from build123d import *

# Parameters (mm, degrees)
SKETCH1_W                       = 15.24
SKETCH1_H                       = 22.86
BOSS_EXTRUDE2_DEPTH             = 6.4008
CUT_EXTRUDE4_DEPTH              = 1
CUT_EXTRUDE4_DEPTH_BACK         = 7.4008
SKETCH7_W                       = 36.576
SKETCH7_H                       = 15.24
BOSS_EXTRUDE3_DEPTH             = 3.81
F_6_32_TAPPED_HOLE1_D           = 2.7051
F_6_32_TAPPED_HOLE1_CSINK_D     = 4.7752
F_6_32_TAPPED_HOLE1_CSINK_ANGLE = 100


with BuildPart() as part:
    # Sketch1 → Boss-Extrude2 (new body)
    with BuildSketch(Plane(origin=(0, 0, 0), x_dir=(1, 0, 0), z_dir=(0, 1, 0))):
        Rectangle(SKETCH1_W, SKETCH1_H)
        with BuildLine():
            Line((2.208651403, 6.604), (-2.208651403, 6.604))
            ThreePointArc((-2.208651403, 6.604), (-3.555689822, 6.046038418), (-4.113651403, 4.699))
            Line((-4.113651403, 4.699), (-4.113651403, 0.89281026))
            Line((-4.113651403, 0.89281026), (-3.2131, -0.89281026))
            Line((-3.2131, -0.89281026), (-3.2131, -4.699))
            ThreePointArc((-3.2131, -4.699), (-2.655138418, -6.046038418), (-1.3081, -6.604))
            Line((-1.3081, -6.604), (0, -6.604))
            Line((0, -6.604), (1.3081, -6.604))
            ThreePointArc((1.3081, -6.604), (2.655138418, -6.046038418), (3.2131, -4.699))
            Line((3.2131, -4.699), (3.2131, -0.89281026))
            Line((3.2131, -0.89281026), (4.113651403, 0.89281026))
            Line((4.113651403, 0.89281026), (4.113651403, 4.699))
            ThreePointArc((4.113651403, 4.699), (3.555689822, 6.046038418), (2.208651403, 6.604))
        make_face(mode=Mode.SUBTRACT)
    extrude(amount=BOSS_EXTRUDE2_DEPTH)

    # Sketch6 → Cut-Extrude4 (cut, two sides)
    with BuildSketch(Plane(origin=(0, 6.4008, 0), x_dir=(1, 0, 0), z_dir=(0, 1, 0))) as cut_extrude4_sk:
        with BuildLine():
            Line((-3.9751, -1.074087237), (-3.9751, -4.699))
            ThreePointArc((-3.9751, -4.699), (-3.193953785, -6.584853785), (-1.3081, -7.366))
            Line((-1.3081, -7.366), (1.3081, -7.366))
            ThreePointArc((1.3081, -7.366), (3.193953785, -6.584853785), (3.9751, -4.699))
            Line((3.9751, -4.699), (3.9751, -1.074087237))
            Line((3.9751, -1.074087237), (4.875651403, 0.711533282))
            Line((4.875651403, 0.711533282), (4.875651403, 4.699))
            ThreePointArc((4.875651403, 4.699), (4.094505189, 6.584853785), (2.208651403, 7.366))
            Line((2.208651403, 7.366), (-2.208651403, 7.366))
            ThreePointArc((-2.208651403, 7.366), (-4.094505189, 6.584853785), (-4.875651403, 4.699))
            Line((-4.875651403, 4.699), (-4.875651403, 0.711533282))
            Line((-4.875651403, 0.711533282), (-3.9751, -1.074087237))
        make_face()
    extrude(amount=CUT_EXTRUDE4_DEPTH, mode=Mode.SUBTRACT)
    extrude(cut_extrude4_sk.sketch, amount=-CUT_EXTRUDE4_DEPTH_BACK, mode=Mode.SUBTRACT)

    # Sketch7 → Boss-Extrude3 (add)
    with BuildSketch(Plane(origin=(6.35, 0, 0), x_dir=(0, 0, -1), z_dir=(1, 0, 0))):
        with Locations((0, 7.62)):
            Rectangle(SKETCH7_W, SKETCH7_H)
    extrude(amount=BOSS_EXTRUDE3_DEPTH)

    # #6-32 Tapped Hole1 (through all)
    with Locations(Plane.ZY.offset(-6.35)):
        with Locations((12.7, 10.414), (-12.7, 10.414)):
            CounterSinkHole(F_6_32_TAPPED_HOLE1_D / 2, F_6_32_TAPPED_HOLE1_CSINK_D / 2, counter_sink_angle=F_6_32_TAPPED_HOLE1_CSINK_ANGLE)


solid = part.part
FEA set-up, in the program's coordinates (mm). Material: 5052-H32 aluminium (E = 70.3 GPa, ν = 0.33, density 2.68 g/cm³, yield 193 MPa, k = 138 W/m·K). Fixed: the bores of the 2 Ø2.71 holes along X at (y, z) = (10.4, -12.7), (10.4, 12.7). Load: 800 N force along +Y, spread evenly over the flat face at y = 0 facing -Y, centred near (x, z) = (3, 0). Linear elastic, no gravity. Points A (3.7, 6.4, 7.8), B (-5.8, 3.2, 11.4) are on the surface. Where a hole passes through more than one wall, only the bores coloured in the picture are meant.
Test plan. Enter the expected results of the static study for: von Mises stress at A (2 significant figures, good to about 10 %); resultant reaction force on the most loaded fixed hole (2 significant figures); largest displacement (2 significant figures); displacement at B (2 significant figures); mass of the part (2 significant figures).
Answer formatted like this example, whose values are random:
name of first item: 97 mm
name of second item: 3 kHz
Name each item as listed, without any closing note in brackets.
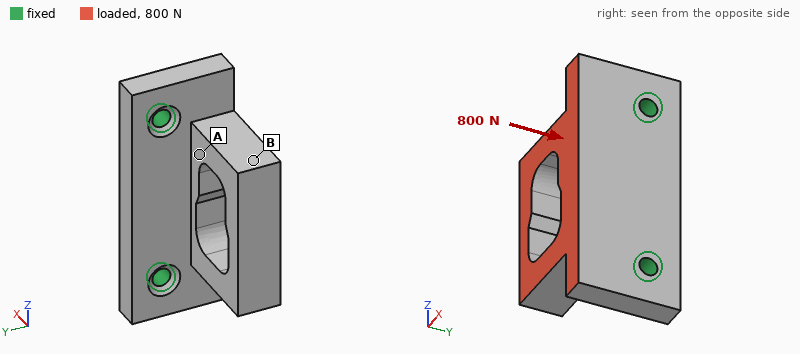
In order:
von Mises stress at A: 45 MPa
resultant reaction force on the most loaded fixed hole: 420 N
largest displacement: 90 µm
displacement at B: 72 µm
mass of the part: 8.9 g
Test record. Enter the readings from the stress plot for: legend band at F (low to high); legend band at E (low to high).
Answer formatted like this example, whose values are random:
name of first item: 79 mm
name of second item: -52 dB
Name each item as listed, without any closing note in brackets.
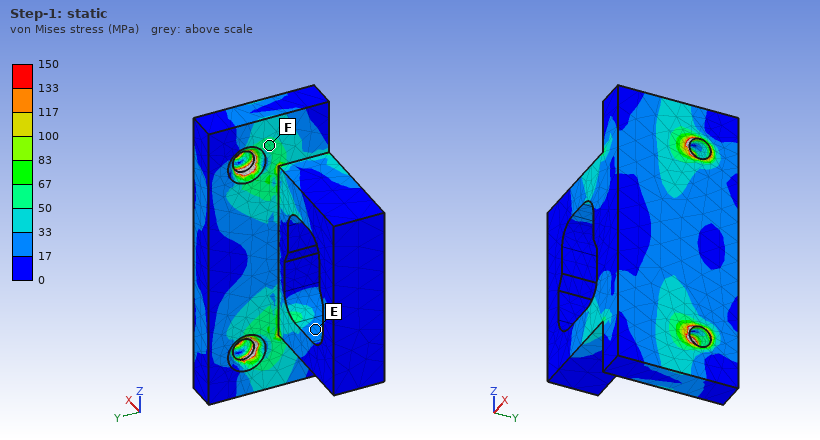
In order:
legend band at F: 50 to 67 MPa
legend band at E: 17 to 33 MPa
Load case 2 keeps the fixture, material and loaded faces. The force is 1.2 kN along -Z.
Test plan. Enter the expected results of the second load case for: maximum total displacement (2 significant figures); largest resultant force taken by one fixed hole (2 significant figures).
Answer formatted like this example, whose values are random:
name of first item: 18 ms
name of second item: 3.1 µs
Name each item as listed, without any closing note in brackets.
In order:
maximum total displacement: 31 µm
largest resultant force taken by one fixed hole: 810 N
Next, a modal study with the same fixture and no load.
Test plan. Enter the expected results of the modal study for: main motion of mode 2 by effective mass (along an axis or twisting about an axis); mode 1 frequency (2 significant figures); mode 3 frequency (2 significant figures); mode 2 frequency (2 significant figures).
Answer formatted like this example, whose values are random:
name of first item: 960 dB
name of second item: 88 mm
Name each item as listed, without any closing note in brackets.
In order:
main motion of mode 2 by effective mass: along Z
mode 1 frequency: 6800 Hz
mode 3 frequency: 19 kHz
mode 2 frequency: 14 kHz
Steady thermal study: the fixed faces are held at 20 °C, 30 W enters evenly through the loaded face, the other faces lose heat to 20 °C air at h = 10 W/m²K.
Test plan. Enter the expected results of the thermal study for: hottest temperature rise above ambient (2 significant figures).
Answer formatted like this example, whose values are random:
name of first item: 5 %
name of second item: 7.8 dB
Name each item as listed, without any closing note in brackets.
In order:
hottest temperature rise above ambient: 37 K
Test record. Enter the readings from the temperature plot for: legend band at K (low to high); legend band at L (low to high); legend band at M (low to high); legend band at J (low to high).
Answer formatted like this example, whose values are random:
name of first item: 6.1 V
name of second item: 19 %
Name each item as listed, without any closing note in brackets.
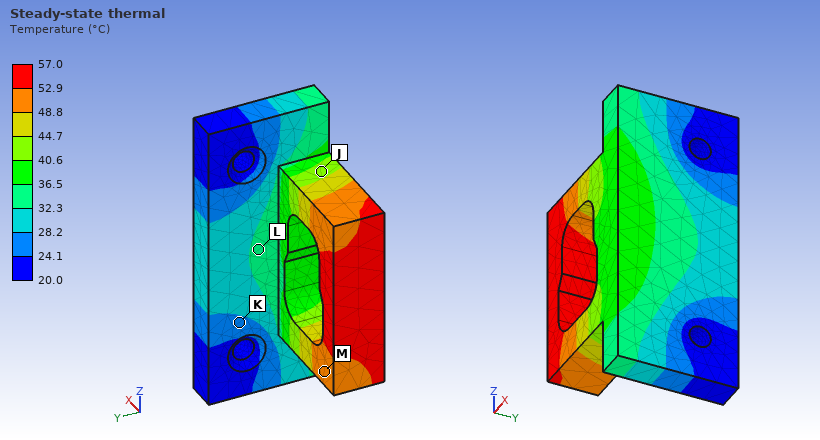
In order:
legend band at K: 24.1 to 28.2 °C
legend band at L: 32.3 to 36.5 °C
legend band at M: 48.8 to 52.9 °C
legend band at J: 40.6 to 44.7 °C
